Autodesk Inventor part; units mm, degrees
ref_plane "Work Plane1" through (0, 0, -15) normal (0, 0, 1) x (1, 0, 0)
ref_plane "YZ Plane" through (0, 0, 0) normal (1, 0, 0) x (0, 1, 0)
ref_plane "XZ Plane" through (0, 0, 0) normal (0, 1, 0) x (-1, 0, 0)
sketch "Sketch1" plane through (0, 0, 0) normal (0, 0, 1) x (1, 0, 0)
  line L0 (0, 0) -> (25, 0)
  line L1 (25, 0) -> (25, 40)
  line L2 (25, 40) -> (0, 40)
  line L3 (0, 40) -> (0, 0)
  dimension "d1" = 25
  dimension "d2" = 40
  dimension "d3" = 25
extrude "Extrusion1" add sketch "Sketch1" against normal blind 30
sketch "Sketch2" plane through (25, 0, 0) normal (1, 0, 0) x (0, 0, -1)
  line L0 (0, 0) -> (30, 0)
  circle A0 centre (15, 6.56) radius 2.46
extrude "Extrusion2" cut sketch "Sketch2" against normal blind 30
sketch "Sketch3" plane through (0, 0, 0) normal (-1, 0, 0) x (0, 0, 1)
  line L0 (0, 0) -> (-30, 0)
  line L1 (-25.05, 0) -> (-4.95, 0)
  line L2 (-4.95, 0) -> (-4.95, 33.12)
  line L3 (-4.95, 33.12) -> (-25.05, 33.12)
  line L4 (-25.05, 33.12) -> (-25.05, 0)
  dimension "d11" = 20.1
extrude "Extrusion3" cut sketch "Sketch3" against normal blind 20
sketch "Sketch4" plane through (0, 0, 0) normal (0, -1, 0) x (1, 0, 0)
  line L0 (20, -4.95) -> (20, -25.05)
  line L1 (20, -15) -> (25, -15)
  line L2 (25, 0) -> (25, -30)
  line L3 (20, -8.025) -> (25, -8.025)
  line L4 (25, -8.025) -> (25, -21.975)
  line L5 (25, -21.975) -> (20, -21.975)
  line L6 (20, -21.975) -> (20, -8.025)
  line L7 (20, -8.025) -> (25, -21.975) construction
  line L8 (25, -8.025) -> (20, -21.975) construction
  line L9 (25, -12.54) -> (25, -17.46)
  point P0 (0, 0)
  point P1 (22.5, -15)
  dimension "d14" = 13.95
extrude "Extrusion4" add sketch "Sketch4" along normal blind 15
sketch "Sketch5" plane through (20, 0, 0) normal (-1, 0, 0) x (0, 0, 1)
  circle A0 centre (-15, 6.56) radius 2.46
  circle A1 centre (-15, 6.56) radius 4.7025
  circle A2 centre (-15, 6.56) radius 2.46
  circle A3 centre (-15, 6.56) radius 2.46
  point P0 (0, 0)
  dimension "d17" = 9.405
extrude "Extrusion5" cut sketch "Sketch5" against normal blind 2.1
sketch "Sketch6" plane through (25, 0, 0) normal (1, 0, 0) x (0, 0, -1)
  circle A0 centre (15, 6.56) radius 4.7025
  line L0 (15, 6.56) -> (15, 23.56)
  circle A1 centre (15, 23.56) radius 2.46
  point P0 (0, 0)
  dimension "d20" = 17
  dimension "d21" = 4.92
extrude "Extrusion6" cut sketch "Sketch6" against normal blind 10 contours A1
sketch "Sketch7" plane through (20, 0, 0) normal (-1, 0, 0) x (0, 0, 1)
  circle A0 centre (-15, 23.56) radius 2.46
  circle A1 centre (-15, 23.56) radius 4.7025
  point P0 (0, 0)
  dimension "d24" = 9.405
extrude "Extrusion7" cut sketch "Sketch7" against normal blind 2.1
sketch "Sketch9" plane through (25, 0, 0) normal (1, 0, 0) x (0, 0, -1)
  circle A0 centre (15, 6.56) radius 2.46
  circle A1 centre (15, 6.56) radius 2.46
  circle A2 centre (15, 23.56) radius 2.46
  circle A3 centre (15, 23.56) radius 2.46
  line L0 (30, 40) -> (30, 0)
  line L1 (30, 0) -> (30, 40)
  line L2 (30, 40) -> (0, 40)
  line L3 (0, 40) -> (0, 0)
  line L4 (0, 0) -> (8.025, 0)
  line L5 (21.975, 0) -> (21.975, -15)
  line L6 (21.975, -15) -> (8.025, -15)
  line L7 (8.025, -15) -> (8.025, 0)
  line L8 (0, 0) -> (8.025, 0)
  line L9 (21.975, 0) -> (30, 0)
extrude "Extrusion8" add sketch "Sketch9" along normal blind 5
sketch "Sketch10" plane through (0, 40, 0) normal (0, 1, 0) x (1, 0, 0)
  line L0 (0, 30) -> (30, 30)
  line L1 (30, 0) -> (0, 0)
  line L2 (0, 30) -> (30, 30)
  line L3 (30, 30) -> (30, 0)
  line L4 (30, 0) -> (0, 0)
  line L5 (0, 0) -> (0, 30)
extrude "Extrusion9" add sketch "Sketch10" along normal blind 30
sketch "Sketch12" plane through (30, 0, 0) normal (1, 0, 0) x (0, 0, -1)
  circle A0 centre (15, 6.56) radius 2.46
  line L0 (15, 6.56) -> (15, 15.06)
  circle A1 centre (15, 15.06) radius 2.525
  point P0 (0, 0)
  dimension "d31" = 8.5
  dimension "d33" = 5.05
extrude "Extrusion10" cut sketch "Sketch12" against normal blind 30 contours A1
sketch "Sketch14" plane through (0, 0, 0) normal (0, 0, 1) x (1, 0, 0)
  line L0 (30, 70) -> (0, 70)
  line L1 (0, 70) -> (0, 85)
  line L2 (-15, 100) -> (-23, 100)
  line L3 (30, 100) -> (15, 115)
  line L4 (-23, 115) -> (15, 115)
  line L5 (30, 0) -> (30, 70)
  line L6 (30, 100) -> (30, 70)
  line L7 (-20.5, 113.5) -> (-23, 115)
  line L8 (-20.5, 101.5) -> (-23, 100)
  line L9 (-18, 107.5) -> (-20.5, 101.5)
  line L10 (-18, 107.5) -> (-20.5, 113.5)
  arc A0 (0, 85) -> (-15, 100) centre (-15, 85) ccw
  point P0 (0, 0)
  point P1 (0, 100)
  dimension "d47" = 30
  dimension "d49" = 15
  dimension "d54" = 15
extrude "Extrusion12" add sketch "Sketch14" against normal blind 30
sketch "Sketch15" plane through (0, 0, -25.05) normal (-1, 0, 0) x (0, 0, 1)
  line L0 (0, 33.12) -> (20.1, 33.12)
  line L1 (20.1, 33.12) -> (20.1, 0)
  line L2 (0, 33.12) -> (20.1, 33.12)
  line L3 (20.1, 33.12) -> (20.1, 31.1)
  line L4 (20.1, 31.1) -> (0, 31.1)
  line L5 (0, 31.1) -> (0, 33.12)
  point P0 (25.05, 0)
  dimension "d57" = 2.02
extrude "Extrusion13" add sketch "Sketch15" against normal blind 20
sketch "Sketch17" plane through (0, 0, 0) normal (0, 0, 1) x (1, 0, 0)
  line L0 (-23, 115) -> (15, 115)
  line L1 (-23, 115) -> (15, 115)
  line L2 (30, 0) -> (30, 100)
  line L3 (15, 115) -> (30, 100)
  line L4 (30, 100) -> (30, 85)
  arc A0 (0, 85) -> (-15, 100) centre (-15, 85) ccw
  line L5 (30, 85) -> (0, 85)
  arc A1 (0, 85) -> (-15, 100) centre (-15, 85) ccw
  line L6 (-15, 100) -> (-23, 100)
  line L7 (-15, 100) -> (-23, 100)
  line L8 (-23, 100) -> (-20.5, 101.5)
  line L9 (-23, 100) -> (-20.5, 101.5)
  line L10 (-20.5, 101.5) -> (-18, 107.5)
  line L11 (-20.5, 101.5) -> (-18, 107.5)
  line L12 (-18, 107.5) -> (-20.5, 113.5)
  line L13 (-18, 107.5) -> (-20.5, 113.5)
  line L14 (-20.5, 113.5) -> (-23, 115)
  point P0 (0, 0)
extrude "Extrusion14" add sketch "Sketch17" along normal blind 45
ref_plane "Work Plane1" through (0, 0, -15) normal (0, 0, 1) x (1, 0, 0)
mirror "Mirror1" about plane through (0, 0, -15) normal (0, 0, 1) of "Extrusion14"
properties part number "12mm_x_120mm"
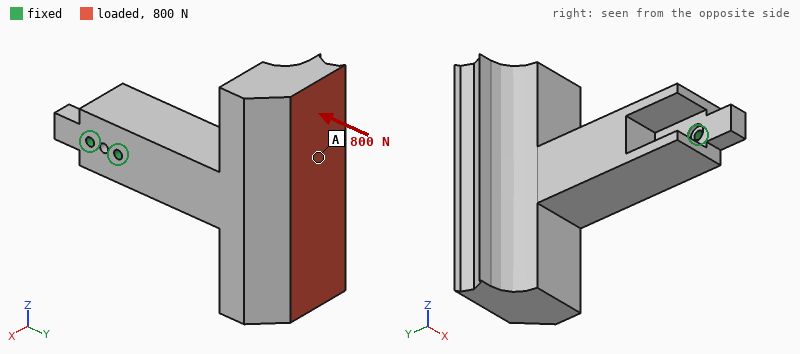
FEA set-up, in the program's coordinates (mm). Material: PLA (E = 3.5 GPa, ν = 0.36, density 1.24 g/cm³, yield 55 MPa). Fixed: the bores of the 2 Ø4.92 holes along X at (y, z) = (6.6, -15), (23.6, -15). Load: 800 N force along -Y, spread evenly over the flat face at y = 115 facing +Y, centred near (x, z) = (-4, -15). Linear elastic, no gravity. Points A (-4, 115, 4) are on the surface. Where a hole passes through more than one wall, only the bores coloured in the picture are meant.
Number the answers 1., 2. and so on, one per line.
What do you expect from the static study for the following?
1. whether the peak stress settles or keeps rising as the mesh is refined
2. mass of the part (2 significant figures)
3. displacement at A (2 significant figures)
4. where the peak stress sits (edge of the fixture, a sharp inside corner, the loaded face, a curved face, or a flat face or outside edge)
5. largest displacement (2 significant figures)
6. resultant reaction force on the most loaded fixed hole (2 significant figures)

1. keeps rising
2. 250 g
3. 1.2 mm
4. edge of the fixture
5. 1.4 mm
6. 1.1 kN
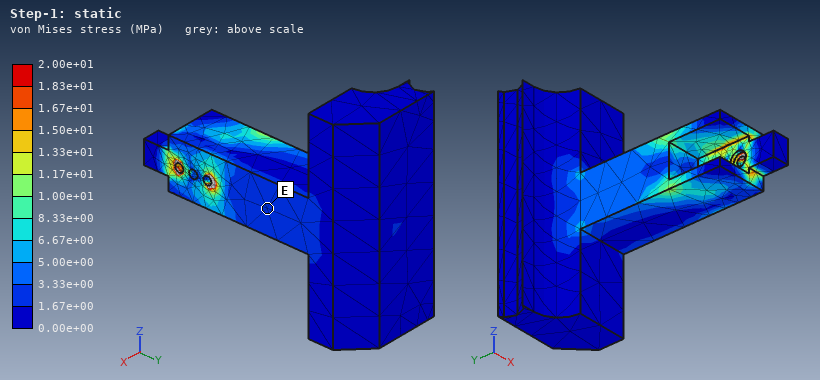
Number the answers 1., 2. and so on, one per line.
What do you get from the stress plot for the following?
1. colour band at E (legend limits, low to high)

1. 1.67e+00 to 3.33e+00 MPa
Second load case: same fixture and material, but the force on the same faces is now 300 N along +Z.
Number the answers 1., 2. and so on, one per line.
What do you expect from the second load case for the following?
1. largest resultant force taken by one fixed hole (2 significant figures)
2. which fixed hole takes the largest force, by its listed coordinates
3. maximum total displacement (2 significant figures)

1. 1.5 kN
2. (23.6, -15)
3. 1.6 mm
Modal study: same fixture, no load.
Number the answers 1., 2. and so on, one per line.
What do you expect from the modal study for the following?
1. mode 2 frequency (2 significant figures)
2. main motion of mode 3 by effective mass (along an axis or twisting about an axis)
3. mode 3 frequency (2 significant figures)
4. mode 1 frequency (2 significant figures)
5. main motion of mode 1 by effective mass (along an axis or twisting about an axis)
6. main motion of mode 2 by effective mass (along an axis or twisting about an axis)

1. 210 Hz
2. twisting about Y
3. 290 Hz
4. 200 Hz
5. along X
6. along Z
